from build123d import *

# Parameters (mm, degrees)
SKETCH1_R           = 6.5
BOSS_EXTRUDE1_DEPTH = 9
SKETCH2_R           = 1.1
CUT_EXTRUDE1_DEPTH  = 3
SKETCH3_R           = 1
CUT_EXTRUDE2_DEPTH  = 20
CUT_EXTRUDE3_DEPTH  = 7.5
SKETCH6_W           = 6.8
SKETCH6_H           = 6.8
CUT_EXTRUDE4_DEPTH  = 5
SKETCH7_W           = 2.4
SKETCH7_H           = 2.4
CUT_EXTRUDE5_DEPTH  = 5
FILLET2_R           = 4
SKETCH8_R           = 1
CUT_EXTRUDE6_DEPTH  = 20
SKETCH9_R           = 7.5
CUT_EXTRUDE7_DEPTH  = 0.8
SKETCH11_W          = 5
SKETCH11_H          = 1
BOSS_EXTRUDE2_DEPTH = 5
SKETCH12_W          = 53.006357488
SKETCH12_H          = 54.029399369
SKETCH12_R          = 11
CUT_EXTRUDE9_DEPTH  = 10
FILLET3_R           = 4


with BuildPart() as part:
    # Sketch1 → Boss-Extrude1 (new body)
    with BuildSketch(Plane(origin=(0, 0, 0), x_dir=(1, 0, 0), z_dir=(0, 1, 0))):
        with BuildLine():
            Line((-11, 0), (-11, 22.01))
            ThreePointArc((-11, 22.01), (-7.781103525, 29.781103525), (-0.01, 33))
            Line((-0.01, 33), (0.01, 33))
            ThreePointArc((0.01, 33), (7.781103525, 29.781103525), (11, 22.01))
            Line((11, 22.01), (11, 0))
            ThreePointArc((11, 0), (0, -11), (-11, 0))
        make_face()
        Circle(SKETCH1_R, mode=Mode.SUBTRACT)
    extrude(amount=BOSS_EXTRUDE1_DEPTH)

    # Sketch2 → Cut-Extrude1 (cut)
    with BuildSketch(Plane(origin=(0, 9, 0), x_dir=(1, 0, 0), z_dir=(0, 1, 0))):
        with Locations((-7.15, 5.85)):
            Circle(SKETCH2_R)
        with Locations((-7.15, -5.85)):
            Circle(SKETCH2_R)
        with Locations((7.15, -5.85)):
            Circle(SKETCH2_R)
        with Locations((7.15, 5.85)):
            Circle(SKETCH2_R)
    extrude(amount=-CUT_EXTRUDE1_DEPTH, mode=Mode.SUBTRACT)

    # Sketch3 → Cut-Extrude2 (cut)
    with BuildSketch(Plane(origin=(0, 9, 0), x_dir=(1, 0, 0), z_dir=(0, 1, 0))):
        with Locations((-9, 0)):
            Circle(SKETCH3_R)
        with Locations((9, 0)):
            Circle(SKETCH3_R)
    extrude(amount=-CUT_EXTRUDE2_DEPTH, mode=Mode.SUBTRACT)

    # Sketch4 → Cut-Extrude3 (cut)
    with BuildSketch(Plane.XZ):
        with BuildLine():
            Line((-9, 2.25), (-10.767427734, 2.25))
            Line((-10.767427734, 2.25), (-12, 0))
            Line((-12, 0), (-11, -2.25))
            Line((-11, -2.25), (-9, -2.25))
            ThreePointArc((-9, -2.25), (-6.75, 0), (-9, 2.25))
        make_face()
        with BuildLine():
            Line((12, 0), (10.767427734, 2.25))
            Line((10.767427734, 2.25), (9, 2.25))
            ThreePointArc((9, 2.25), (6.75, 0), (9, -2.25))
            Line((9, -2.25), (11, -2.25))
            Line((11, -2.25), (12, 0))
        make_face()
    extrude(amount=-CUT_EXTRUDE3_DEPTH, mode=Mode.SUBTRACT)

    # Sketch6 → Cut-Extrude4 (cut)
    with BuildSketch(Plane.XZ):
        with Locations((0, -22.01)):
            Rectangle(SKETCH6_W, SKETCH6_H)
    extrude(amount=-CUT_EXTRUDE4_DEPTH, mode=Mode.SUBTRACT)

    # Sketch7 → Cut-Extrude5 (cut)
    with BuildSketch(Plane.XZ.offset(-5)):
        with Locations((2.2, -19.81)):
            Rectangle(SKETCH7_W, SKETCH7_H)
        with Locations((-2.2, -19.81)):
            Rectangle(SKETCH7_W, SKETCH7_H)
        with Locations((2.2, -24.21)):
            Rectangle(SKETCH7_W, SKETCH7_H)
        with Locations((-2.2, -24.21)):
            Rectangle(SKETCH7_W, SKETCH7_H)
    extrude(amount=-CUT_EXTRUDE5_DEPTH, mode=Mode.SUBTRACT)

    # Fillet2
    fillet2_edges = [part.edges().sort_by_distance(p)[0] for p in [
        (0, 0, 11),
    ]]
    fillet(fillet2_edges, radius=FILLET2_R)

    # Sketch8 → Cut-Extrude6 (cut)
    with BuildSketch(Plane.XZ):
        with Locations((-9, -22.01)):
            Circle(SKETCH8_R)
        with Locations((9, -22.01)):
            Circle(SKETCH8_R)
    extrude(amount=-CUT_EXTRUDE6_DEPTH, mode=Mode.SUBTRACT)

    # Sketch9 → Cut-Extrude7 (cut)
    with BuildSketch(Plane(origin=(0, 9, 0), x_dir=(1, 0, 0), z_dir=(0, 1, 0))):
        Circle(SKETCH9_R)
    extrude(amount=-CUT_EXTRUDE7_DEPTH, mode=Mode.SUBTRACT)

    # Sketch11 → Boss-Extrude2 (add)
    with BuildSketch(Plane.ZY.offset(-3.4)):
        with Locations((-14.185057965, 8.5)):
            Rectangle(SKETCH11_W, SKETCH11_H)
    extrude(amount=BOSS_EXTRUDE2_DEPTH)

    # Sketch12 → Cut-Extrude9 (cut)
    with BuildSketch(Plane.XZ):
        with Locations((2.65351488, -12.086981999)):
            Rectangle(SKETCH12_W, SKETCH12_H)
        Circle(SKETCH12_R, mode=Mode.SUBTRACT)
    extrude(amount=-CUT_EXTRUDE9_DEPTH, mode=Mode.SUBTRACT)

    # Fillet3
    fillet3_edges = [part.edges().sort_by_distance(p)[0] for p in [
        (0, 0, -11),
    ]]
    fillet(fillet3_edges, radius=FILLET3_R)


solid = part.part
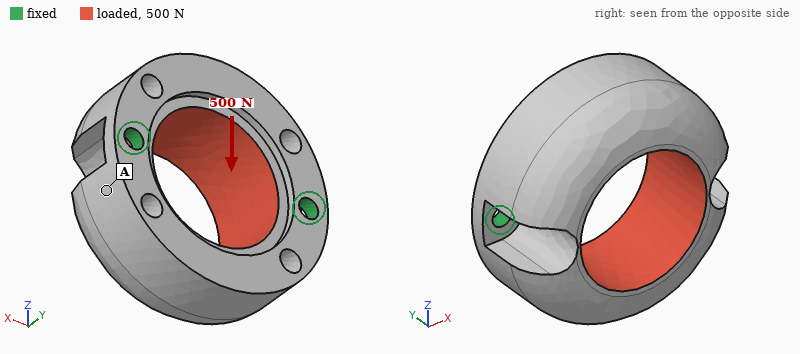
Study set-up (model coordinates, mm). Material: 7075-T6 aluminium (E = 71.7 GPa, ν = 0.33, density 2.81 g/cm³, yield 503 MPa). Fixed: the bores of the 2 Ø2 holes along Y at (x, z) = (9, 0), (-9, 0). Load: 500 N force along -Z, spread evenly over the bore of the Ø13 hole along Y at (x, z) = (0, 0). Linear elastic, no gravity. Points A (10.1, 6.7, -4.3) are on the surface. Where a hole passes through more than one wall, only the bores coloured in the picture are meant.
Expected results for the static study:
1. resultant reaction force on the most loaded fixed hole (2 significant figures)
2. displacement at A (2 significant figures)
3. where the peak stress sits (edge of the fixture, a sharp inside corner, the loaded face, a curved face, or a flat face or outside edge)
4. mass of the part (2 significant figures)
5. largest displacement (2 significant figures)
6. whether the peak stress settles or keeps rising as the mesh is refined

250 N
22 µm
edge of the fixture
4.8 g
71 µm
keeps rising
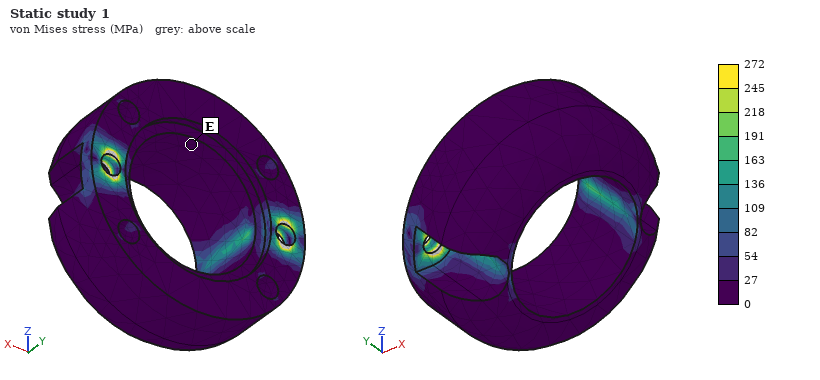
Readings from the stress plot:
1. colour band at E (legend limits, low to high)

0 to 27 MPa
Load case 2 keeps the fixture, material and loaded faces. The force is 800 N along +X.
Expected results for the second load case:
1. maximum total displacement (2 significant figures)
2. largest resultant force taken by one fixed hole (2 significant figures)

13 µm
440 N
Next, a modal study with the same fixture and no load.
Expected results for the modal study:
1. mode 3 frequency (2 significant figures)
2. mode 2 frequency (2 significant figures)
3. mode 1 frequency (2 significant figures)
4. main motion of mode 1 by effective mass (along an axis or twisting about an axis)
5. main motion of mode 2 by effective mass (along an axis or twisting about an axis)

23 kHz
21 kHz
5800 Hz
along Z
along Y
